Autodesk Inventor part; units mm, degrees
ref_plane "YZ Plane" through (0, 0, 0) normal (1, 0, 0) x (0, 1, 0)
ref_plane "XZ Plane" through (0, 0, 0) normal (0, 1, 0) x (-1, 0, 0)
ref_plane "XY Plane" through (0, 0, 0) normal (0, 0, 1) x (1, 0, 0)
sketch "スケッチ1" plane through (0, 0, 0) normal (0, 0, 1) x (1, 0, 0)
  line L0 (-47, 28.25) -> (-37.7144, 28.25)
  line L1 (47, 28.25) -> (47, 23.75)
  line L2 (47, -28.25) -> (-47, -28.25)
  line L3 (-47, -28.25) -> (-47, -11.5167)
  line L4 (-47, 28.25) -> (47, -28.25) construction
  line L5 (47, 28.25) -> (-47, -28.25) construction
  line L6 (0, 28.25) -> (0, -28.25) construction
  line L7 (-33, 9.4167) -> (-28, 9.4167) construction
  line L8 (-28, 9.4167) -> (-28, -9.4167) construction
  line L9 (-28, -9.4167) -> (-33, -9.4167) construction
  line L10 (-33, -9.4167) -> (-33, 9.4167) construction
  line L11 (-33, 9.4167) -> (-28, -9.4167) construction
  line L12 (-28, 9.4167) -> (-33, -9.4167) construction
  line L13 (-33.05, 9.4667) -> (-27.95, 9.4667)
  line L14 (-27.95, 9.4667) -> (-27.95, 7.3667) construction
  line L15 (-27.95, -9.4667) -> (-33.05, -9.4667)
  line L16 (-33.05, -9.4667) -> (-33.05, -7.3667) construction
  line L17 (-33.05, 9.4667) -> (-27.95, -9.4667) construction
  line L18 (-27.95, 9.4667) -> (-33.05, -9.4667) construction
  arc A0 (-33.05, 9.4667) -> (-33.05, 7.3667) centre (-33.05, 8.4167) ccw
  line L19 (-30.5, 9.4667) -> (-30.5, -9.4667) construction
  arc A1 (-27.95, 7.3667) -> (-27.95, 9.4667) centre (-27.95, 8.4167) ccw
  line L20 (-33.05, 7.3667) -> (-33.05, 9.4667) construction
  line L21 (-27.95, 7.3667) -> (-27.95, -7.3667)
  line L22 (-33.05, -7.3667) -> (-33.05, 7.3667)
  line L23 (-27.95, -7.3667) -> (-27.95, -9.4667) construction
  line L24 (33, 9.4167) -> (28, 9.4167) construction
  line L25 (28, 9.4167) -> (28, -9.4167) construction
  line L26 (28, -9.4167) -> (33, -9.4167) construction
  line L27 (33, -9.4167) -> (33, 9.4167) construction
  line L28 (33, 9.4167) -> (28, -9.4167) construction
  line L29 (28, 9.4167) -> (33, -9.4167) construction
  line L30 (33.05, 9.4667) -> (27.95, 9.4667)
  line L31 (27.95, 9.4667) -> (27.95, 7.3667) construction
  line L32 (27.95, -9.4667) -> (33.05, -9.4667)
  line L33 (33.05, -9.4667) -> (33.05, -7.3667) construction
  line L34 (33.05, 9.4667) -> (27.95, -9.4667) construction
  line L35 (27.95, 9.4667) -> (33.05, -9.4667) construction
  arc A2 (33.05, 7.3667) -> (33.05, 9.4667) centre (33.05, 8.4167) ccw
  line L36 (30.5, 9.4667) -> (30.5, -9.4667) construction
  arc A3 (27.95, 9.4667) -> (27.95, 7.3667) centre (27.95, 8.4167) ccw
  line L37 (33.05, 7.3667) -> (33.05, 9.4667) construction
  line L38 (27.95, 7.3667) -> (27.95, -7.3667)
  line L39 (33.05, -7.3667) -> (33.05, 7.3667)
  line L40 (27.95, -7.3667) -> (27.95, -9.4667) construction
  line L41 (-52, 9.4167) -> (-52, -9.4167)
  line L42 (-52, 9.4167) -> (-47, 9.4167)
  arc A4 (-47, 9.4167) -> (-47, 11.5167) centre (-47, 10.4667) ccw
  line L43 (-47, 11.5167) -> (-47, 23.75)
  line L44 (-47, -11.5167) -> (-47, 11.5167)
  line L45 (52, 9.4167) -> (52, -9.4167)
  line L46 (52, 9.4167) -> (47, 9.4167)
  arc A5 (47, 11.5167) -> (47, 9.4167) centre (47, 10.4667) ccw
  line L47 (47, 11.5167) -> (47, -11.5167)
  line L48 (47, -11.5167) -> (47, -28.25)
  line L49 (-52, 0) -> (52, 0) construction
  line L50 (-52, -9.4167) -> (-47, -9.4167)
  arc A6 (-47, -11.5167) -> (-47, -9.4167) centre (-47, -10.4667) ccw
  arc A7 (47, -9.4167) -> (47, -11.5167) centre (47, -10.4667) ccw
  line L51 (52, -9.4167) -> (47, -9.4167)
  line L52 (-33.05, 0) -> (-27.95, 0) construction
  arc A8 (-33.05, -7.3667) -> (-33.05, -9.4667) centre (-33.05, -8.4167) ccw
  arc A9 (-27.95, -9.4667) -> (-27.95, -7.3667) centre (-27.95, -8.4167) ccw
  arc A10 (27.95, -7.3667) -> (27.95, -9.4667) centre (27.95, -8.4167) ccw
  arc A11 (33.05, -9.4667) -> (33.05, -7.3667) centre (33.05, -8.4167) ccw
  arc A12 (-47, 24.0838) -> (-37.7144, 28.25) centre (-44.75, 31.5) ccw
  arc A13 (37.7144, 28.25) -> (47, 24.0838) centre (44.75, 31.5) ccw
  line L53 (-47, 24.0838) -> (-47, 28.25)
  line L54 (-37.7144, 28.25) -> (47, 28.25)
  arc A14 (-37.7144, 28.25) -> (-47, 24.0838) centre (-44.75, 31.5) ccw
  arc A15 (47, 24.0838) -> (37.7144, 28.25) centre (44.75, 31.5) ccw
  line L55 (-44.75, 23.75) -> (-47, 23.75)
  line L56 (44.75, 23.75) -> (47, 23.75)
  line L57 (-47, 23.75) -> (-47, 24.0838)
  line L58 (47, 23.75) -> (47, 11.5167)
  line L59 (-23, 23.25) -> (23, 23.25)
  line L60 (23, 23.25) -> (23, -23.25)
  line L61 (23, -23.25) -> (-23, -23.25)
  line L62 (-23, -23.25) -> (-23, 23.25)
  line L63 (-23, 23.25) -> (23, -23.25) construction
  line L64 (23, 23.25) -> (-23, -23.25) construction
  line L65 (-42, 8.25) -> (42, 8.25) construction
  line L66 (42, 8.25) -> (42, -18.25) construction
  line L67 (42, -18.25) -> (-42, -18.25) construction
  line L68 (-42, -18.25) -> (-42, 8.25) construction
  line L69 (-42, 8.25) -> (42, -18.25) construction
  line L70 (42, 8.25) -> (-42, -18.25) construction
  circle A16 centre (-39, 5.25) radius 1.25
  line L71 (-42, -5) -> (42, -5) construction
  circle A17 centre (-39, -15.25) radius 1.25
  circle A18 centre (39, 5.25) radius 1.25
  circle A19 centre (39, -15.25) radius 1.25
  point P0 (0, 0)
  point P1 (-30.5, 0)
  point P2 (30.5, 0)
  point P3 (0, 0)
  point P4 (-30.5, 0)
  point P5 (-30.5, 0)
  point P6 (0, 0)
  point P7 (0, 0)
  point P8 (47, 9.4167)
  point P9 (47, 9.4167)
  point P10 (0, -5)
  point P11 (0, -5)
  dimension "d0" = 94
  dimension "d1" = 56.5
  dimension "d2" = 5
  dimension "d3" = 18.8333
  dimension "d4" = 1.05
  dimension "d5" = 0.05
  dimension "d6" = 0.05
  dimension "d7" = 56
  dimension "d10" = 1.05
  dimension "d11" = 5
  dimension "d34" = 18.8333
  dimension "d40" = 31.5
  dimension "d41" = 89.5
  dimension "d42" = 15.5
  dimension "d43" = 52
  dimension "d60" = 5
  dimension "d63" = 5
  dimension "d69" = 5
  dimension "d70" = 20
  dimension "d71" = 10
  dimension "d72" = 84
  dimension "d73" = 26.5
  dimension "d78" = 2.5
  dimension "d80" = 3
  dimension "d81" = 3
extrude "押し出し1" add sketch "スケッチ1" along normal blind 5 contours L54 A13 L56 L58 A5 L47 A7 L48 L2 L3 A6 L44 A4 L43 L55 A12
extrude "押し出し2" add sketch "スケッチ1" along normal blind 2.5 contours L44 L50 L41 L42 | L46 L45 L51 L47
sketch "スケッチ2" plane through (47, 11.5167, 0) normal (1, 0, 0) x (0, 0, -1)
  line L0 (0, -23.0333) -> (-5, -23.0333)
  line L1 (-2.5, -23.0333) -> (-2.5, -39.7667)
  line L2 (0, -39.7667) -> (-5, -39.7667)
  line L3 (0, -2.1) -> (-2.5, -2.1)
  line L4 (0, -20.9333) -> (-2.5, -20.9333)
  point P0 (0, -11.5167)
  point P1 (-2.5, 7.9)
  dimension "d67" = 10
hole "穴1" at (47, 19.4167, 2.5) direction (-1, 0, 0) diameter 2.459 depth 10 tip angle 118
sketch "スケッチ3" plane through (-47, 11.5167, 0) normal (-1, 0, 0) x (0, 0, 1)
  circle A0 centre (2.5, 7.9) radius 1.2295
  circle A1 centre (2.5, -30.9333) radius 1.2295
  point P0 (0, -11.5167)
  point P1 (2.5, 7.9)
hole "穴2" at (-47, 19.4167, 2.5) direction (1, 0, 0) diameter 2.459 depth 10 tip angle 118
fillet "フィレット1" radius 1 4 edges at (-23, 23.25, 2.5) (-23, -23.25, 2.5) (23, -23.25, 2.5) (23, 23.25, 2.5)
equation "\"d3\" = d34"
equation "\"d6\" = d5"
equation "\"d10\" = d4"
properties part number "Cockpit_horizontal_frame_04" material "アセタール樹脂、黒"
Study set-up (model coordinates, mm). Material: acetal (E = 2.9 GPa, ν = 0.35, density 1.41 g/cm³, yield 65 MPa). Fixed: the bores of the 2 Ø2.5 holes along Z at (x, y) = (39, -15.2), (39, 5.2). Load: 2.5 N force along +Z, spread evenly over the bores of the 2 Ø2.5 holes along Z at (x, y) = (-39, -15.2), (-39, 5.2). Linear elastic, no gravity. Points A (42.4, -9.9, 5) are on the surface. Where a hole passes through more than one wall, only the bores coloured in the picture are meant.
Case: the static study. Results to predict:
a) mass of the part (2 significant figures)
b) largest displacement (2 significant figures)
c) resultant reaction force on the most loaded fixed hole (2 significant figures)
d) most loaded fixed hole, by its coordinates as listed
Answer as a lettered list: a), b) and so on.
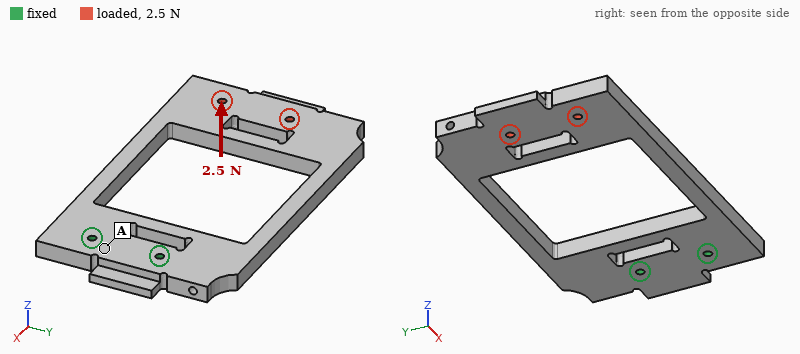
a) 21 g
b) 1.3 mm
c) 2.2 N
d) (39, -15.2)
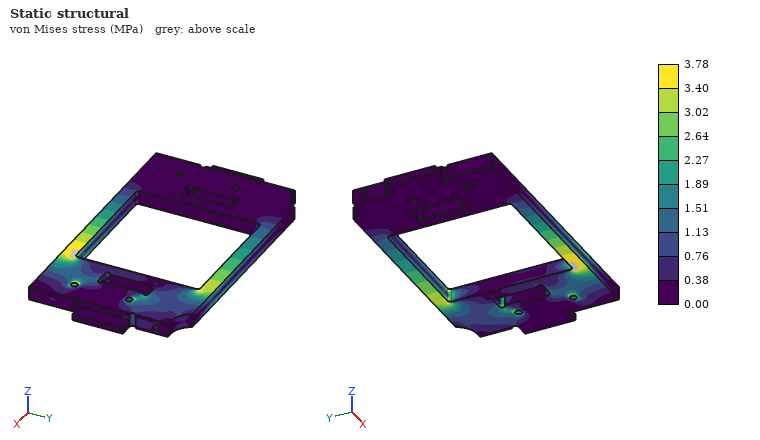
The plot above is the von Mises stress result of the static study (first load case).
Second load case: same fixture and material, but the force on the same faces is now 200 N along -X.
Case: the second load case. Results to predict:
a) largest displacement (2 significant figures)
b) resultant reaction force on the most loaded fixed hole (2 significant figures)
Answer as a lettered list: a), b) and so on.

a) 0.17 mm
b) 110 N
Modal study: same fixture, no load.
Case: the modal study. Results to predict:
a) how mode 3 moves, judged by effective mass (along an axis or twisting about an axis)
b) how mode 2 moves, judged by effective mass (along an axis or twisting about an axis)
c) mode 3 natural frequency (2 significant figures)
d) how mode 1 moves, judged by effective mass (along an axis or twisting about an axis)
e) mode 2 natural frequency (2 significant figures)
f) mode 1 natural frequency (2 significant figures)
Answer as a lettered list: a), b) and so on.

a) twisting about X
b) along Y
c) 290 Hz
d) along Z
e) 240 Hz
f) 86 Hz
